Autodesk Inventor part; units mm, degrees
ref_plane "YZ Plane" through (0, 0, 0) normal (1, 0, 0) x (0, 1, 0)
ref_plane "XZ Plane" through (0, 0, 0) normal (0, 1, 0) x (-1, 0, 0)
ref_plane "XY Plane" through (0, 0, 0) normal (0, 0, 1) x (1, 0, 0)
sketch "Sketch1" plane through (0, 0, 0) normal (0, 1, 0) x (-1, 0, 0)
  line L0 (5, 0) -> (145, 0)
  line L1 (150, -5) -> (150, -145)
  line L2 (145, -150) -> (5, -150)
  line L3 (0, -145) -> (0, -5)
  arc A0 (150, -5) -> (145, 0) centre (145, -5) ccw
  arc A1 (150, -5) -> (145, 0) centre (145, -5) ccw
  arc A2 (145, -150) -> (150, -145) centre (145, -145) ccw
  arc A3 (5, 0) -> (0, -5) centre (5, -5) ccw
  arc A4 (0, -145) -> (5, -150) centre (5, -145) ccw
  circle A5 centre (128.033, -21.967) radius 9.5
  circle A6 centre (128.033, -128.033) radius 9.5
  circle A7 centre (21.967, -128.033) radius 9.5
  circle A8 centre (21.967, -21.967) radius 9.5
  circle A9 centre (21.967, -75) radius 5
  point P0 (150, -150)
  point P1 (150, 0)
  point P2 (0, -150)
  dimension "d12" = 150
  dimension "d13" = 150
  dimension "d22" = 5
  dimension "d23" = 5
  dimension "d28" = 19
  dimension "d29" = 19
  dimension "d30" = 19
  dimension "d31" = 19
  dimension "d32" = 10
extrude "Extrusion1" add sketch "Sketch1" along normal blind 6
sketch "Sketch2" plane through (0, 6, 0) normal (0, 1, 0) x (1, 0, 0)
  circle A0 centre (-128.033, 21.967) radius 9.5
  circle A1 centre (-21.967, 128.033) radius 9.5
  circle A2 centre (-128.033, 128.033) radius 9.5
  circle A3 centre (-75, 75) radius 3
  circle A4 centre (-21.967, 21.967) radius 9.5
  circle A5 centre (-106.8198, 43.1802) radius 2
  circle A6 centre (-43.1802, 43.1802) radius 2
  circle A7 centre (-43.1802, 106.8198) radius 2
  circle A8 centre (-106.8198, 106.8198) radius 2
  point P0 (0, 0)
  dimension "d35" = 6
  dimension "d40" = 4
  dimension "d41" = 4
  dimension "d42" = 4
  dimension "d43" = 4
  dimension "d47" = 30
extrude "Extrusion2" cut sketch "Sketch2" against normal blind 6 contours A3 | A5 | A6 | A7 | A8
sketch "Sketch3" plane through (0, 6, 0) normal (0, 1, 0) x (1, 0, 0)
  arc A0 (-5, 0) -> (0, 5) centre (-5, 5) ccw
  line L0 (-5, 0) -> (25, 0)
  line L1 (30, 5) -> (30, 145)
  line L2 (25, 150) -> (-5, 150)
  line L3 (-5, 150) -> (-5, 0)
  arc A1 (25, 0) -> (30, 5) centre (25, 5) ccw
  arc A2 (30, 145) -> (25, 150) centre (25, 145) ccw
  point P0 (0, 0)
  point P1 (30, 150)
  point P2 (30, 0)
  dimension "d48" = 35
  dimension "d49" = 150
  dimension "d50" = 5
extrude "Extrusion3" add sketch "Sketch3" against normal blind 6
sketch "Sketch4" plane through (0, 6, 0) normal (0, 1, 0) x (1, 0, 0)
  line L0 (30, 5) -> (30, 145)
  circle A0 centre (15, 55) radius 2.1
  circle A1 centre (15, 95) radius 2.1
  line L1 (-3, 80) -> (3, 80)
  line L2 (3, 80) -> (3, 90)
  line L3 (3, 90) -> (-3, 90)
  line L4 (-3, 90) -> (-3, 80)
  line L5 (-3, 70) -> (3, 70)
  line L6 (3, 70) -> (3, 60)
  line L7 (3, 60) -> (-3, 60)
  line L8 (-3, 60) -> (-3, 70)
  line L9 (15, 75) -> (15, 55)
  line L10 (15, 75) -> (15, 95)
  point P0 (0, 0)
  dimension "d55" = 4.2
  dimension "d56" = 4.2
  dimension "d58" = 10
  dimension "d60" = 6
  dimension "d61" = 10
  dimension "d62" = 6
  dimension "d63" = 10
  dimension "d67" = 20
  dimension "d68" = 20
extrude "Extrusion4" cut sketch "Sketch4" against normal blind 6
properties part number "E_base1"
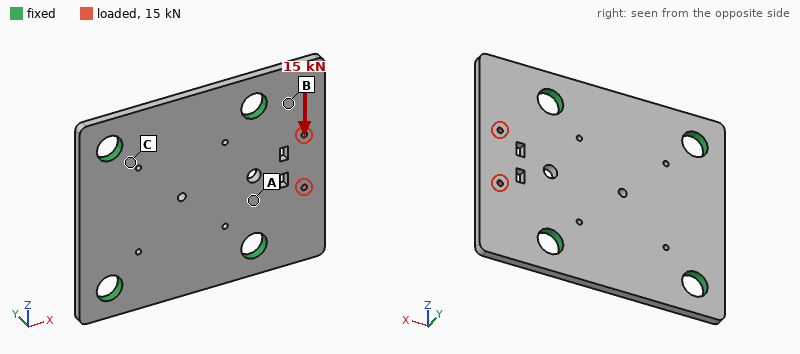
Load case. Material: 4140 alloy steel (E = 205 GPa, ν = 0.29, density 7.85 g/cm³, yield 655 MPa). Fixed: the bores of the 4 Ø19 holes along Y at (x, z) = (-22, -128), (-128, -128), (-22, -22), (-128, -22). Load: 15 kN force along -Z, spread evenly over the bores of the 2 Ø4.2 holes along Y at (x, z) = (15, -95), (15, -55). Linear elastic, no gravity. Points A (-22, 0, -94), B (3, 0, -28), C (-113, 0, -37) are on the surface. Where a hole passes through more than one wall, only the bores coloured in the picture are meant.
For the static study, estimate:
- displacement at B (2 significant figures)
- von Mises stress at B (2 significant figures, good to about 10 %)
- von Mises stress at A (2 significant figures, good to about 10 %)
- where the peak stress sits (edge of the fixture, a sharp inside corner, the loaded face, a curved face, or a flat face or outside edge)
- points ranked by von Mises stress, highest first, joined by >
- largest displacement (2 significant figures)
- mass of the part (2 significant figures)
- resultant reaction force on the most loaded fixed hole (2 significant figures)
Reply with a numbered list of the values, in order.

1. 6.2 µm
2. 31 MPa
3. 20 MPa
4. the loaded face
5. B > A > C
6. 15 µm
7. 1.2 kg
8. 8.5 kN
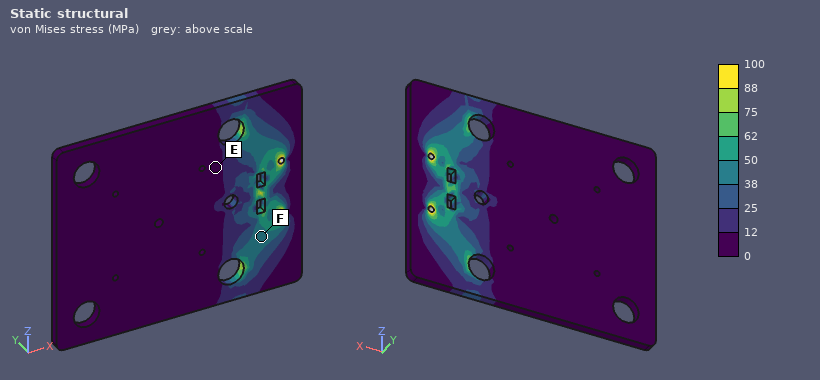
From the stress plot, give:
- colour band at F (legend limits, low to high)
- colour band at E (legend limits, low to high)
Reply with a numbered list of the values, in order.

1. 38 to 50 MPa
2. 0 to 12 MPa
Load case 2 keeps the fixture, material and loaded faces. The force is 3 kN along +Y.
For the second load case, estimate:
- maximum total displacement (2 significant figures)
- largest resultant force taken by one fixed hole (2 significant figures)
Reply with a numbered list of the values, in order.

1. 0.23 mm
2. 1.6 kN
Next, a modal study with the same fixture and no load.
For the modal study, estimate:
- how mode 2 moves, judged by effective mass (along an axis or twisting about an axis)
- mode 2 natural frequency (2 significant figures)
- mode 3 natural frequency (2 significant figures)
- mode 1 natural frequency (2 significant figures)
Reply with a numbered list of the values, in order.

1. along Y
2. 2500 Hz
3. 2900 Hz
4. 1900 Hz
